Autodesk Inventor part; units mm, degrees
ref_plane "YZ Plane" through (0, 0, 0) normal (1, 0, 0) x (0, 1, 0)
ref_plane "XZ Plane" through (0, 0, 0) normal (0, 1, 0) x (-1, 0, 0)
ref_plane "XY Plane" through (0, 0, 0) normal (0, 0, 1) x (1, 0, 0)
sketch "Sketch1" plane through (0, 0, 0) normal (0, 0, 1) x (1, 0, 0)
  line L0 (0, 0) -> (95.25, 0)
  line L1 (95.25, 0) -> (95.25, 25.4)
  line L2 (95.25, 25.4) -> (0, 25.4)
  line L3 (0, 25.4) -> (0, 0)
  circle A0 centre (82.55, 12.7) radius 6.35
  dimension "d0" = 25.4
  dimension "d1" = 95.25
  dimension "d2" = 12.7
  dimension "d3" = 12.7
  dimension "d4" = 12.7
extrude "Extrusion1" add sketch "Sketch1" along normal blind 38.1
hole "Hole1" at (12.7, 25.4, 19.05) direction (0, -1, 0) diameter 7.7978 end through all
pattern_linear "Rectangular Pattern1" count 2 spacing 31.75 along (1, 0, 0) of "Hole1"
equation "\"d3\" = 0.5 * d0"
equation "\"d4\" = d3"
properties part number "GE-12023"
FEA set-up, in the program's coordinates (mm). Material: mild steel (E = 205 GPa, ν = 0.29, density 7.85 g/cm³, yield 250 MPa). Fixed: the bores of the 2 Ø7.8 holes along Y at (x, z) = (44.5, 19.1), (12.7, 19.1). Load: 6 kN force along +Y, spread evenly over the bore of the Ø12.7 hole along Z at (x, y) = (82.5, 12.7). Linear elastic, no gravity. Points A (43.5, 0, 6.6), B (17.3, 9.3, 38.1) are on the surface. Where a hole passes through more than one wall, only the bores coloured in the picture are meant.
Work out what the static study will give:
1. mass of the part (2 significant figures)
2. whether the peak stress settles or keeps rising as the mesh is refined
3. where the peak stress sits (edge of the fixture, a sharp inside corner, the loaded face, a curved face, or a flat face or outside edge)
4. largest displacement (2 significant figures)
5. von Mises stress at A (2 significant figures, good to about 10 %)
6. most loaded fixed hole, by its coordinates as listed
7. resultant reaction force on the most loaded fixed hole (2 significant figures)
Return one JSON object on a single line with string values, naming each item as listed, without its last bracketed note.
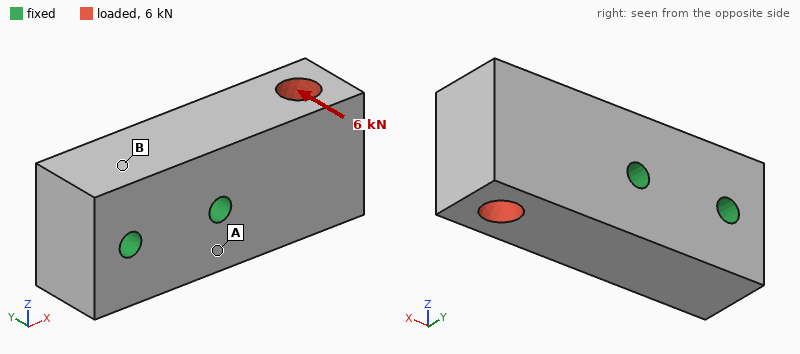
{"mass of the part": "670 g", "whether the peak stress settles or keeps rising as the mesh is refined": "keeps rising", "where the peak stress sits": "edge of the fixture", "largest displacement": "25 µm", "von Mises stress at A": "29 MPa", "most loaded fixed hole, by its coordinates as listed": "(44.5, 19.1)", "resultant reaction force on the most loaded fixed hole": "7.6 kN"}
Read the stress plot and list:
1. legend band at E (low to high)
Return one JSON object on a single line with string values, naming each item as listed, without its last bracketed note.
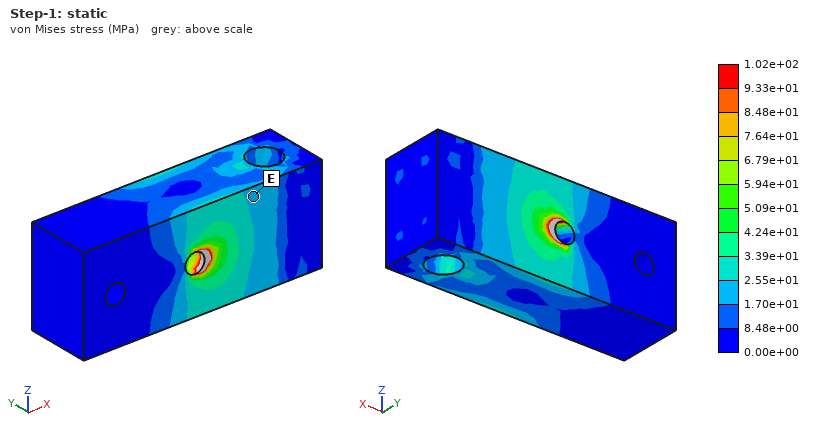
{"legend band at E": "1.70e+01 to 2.55e+01 MPa"}
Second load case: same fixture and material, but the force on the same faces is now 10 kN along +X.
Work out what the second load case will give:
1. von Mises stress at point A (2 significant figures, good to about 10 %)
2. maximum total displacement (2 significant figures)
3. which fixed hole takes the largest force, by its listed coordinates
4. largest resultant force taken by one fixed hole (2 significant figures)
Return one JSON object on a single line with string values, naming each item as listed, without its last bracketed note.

{"von Mises stress at point A": "6.0 MPa", "maximum total displacement": "3.6 µm", "which fixed hole takes the largest force, by its listed coordinates": "(44.5, 19.1)", "largest resultant force taken by one fixed hole": "8.3 kN"}
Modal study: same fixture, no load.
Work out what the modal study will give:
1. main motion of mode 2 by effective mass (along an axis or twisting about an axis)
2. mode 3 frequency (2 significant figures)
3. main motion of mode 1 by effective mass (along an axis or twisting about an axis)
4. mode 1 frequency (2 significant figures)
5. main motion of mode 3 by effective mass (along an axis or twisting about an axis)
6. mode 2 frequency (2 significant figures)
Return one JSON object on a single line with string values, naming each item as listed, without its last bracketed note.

{"main motion of mode 2 by effective mass": "along Z", "mode 3 frequency": "13 kHz", "main motion of mode 1 by effective mass": "along Y", "mode 1 frequency": "6800 Hz", "main motion of mode 3 by effective mass": "twisting about X", "mode 2 frequency": "7300 Hz"}
